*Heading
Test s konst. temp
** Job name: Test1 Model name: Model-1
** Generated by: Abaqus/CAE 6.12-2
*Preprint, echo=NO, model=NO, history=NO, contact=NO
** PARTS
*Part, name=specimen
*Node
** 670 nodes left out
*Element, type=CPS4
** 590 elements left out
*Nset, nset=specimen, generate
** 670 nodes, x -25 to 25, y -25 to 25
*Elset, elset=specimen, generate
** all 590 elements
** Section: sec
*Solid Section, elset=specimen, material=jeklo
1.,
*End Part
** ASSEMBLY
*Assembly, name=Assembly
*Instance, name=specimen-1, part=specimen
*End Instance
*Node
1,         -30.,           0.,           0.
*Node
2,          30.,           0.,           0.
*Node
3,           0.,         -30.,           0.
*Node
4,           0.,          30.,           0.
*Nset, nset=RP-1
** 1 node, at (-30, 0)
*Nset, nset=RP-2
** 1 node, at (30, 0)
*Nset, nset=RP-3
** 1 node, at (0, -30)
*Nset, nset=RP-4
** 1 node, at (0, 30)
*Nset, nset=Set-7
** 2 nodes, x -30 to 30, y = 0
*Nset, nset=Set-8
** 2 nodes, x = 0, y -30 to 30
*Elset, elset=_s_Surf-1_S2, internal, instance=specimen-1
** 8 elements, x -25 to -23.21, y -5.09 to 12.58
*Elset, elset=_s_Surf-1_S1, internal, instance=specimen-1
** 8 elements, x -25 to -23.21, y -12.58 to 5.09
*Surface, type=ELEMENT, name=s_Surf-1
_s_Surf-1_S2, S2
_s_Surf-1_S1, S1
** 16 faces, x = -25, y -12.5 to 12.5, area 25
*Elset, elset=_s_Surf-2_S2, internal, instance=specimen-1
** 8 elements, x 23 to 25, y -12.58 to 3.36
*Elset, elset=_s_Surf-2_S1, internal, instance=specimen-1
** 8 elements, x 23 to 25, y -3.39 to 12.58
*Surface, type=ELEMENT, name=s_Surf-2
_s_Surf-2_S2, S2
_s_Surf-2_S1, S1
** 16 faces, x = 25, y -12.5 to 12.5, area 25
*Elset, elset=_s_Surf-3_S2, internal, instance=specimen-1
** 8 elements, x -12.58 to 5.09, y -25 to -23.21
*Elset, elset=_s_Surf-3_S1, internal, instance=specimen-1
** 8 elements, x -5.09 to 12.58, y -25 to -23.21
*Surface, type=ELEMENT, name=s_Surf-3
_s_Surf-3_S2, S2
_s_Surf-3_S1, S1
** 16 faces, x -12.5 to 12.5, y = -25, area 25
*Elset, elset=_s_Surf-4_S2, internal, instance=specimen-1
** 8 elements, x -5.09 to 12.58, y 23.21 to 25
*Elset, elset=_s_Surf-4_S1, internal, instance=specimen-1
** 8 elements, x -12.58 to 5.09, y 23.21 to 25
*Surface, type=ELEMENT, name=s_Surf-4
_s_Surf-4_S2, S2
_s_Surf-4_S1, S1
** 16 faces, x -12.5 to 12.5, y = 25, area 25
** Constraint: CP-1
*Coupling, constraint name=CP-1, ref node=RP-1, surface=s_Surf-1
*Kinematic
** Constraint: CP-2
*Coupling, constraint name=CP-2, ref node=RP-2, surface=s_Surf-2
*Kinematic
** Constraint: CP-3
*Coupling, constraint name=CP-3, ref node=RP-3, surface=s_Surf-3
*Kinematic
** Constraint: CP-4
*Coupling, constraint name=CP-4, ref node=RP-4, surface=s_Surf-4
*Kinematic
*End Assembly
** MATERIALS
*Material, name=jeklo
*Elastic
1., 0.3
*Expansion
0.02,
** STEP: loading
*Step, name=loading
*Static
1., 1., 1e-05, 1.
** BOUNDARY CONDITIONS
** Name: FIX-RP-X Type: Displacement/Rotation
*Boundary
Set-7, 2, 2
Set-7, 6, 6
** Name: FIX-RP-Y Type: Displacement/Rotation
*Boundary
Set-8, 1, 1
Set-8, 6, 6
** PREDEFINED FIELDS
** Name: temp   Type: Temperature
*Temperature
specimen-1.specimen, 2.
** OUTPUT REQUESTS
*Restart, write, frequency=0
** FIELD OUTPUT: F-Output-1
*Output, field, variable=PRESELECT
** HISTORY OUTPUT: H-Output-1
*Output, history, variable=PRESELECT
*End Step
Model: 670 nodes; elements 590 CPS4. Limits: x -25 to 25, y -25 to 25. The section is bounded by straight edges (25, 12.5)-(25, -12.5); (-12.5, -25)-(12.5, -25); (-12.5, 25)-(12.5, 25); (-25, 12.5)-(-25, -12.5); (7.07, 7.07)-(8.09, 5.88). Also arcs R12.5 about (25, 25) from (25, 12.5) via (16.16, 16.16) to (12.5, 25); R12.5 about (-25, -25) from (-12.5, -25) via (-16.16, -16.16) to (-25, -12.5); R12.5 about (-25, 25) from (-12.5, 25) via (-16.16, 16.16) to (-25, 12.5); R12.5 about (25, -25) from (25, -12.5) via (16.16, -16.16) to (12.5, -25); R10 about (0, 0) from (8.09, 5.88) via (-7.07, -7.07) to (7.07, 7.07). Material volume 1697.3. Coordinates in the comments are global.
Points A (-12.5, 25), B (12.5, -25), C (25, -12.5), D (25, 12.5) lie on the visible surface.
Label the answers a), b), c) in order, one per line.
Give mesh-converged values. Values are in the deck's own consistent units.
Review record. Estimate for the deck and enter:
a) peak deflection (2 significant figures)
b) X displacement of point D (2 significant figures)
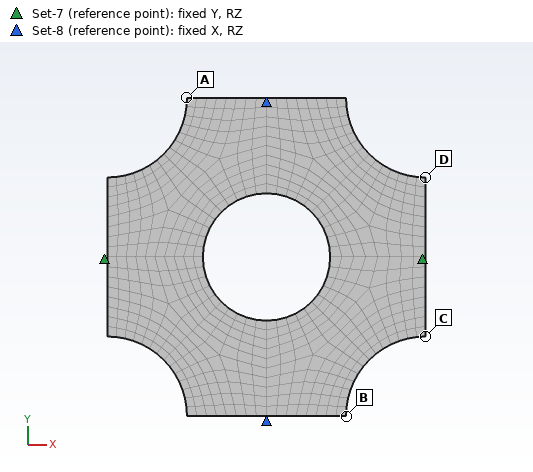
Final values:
a) 1.0
b) 0.97
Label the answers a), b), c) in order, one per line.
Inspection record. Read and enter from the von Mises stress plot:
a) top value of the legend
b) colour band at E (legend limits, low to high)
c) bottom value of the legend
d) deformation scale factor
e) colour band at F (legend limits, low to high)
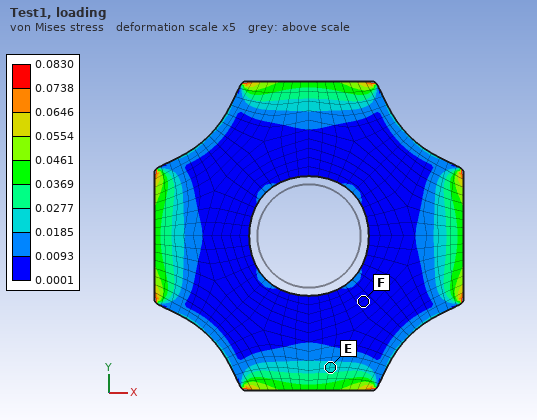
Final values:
a) 0.0830
b) 0.0185 to 0.0277
c) 0.0001
d) 5
e) 0.0001 to 0.0093
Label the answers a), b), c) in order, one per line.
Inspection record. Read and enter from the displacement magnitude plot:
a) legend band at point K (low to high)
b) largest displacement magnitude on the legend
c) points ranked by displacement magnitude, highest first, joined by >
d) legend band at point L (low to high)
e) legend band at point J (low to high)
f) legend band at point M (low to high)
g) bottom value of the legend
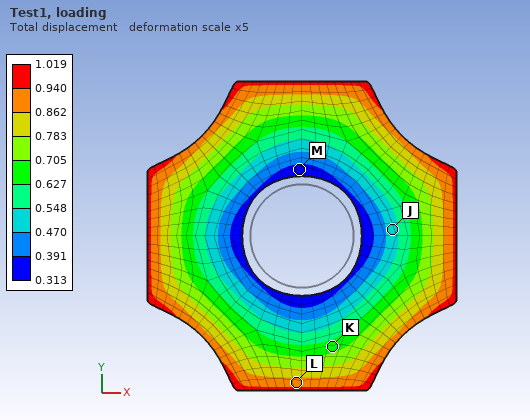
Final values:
a) 0.627 to 0.705
b) 1.019
c) L > K > J > M
d) 0.862 to 0.940
e) 0.470 to 0.548
f) 0.313 to 0.391
g) 0.313
